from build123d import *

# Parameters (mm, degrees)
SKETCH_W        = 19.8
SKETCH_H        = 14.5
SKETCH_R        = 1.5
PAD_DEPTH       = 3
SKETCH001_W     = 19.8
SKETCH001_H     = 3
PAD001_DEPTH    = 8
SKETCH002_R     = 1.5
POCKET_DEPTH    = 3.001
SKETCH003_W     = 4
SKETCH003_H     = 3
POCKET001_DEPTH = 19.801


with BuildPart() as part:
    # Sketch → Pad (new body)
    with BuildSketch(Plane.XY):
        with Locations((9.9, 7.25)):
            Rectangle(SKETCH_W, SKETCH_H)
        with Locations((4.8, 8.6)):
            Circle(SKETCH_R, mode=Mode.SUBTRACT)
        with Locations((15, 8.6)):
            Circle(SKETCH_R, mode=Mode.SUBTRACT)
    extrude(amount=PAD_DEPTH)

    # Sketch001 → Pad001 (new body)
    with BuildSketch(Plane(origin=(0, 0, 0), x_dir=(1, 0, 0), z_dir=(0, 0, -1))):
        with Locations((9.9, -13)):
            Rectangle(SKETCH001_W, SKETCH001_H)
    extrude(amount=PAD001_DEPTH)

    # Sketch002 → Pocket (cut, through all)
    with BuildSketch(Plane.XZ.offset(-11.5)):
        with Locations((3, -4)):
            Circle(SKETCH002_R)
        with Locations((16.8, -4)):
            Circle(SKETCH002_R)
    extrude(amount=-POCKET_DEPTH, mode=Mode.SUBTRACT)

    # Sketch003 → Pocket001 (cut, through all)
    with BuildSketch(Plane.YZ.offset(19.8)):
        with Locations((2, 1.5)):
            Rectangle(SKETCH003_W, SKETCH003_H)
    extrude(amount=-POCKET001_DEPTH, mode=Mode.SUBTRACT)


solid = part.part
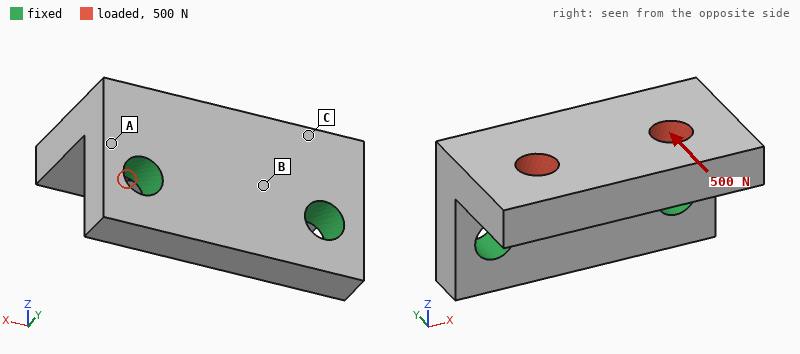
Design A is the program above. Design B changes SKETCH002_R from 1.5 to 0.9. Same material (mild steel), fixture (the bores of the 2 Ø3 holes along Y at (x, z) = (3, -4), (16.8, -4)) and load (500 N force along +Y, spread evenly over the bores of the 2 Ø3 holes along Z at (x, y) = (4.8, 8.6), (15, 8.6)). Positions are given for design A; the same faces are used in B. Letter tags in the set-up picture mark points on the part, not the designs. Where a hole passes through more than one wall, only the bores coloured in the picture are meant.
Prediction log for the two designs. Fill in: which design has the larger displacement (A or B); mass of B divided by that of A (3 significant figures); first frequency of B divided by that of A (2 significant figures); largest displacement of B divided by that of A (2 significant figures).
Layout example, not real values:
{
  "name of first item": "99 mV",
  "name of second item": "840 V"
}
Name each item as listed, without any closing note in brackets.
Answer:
{
  "which design has the larger displacement": "B",
  "mass of B divided by that of A": "1.03",
  "first frequency of B divided by that of A": "0.89",
  "largest displacement of B divided by that of A": "1.4"
}
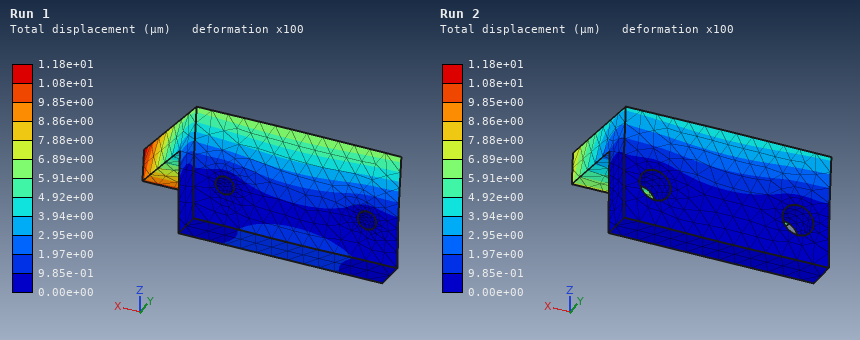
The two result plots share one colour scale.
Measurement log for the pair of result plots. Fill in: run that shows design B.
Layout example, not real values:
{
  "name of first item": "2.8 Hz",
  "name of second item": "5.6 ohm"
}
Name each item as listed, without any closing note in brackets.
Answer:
{
  "run that shows design B": "Run 1"
}
